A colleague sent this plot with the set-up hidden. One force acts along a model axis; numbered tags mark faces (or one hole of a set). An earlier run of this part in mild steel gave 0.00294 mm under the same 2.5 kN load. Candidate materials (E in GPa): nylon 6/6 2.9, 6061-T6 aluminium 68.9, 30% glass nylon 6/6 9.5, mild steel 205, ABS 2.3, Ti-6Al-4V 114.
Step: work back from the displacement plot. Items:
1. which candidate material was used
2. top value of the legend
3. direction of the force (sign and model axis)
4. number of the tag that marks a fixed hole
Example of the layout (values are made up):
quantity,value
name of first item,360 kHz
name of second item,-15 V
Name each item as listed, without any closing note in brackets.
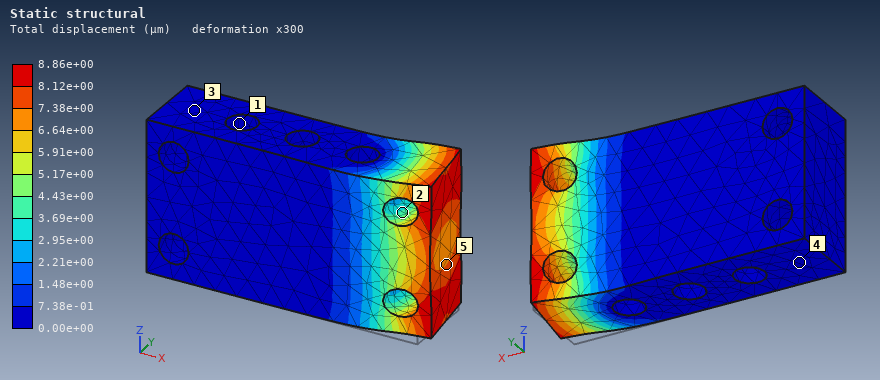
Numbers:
quantity,value
which candidate material was used,6061-T6 aluminium
top value of the legend,8.86e+00 µm
direction of the force,+Y
number of the tag that marks a fixed hole,1
